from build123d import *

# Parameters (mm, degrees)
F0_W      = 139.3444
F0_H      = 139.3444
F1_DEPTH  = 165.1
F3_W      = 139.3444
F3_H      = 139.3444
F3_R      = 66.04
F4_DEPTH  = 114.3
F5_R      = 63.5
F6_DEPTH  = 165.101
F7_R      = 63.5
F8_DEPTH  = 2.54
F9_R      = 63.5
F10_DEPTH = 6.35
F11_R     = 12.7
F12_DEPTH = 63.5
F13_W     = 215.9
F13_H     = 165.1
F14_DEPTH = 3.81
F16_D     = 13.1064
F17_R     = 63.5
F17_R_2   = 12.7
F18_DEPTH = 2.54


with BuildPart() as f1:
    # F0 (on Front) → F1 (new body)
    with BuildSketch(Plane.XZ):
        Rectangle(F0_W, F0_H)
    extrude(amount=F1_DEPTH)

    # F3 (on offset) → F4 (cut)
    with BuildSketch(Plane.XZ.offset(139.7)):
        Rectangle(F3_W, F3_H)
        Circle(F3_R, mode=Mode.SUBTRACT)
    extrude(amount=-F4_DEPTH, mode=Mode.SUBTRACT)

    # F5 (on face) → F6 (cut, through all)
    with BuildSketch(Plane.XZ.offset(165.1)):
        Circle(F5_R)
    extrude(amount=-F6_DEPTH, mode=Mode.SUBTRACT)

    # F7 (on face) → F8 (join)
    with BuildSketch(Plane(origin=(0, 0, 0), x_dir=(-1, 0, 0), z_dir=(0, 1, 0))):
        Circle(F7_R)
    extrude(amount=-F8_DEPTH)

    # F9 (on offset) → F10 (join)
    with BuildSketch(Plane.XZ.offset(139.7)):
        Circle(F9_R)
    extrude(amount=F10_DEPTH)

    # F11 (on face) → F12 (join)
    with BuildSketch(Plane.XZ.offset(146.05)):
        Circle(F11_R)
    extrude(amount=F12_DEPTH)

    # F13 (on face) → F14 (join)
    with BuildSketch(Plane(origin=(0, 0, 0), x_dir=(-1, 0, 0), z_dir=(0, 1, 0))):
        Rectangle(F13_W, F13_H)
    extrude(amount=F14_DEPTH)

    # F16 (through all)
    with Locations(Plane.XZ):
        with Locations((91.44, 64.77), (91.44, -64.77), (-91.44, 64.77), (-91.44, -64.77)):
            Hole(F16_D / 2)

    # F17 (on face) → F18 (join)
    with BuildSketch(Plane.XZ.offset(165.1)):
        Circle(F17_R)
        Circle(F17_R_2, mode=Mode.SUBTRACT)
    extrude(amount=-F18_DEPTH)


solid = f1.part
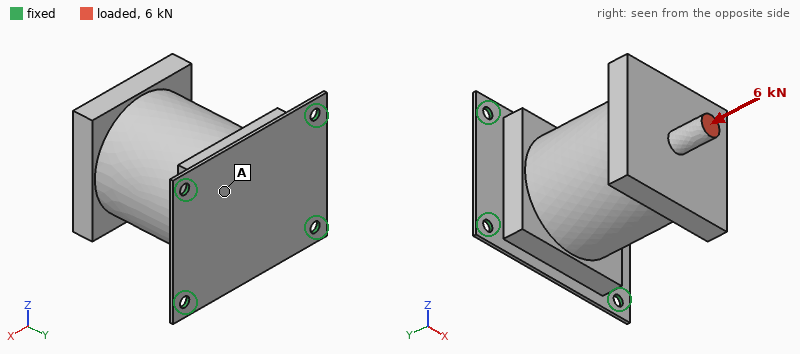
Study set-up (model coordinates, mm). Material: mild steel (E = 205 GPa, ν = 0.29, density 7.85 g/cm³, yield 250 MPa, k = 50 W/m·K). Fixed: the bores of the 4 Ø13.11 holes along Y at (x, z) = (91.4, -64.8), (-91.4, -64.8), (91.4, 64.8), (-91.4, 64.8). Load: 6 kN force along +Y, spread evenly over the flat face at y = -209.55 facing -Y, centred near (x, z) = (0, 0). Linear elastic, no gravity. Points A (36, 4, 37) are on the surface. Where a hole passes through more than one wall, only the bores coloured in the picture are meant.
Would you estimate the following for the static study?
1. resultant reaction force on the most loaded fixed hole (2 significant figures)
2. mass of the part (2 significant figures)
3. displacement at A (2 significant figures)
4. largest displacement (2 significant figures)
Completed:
2.0 kN
6.0 kg
0.038 mm
0.11 mm
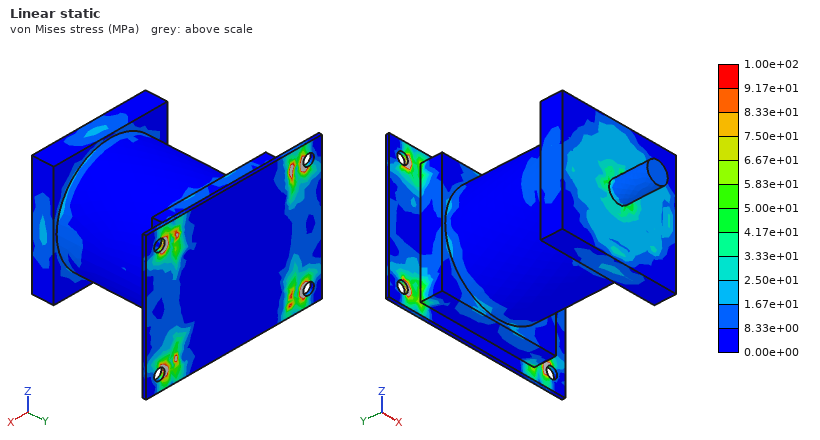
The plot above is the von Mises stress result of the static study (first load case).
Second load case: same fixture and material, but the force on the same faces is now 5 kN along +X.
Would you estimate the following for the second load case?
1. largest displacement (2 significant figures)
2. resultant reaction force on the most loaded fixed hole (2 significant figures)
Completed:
0.41 mm
3.9 kN
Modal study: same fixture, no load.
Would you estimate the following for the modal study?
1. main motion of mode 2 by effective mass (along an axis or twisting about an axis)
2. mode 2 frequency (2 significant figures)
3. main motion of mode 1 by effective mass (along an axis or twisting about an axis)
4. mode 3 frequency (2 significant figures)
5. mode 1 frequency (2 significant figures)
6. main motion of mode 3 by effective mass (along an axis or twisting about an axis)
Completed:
along X
520 Hz
along Z
830 Hz
410 Hz
along Y
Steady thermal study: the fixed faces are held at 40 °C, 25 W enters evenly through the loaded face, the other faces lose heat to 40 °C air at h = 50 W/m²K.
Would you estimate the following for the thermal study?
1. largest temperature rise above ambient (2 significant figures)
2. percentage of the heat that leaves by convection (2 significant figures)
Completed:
55 K
100 %
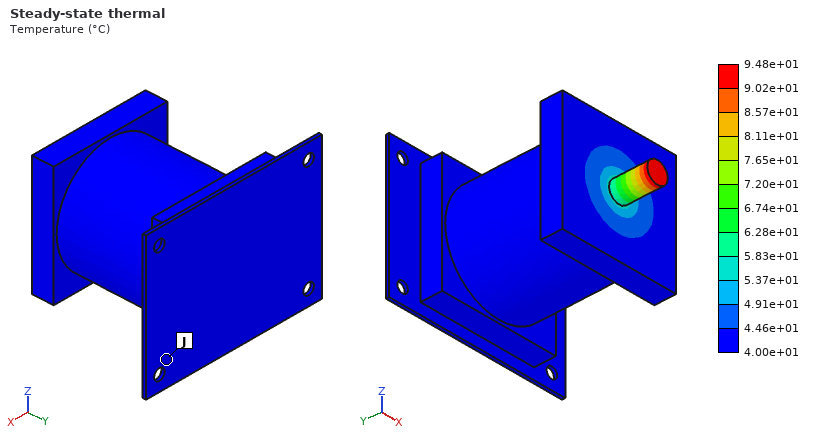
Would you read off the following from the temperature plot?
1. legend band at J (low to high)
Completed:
4.00e+01 to 4.46e+01 °C
